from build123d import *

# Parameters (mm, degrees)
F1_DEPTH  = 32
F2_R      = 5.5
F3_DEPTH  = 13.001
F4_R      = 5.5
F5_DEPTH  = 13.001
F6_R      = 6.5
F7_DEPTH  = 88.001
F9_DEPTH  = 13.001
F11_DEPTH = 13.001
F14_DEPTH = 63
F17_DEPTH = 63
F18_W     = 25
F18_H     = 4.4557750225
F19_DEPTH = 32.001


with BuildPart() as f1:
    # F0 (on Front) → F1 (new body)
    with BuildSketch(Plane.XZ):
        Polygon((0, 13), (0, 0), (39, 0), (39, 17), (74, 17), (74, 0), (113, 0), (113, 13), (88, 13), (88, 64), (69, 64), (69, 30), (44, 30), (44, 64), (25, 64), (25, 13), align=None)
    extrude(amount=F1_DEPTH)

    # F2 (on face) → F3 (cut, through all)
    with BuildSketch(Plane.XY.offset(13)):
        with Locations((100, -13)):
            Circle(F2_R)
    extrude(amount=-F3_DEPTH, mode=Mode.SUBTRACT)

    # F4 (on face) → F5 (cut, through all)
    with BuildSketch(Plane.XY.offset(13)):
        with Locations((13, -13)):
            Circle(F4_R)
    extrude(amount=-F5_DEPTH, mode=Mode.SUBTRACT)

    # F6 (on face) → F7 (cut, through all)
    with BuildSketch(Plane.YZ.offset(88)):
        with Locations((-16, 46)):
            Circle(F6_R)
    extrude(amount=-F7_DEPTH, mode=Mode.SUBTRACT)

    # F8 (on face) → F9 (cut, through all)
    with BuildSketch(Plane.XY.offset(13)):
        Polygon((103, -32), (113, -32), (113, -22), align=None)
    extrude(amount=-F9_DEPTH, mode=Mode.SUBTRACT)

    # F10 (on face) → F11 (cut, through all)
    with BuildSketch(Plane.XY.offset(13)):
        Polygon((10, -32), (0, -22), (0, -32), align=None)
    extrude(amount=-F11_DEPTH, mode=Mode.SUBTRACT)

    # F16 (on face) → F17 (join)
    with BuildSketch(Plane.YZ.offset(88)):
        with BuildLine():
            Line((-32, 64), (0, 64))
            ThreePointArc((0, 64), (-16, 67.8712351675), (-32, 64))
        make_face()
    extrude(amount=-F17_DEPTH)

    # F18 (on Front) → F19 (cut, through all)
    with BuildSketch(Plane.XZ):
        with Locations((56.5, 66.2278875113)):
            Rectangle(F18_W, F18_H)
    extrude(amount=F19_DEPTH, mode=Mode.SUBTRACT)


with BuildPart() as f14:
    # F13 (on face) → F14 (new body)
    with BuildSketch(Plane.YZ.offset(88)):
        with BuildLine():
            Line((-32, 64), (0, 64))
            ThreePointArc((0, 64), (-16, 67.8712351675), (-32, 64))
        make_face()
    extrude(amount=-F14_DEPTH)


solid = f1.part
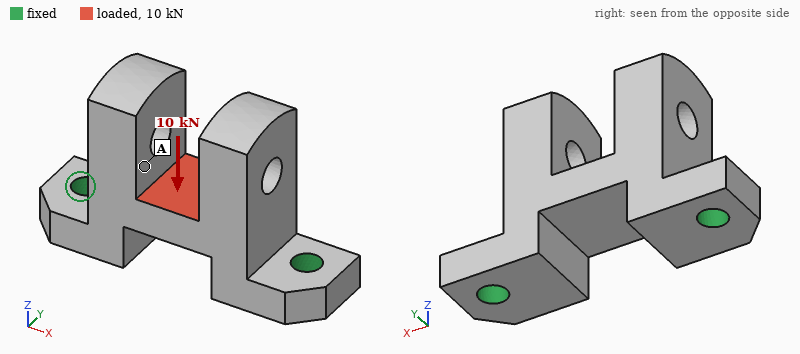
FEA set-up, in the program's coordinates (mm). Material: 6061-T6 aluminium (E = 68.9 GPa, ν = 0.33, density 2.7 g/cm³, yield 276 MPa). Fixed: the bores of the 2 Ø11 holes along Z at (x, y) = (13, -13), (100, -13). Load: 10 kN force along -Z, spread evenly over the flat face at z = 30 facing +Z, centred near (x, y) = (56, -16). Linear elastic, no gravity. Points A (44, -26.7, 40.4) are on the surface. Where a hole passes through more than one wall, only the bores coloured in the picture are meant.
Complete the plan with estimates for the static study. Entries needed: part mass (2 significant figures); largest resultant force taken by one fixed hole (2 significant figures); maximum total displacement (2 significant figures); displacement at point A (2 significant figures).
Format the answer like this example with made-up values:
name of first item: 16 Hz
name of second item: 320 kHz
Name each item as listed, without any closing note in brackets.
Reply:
part mass: 260 g
largest resultant force taken by one fixed hole: 7.4 kN
maximum total displacement: 54 µm
displacement at point A: 37 µm
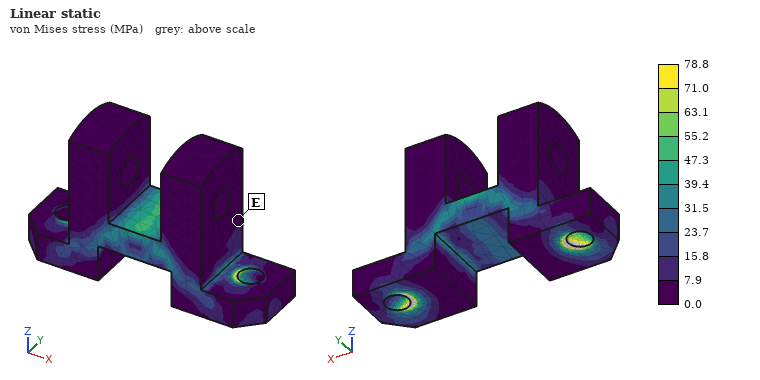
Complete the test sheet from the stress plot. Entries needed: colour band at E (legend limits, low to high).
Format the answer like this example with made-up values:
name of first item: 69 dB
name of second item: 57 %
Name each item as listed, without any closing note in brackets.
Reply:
colour band at E: 0.0 to 7.9 MPa
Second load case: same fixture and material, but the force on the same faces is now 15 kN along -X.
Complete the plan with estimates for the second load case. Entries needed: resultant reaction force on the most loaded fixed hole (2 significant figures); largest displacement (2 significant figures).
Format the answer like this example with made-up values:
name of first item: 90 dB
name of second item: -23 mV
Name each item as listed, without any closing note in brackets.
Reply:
resultant reaction force on the most loaded fixed hole: 8.7 kN
largest displacement: 41 µm
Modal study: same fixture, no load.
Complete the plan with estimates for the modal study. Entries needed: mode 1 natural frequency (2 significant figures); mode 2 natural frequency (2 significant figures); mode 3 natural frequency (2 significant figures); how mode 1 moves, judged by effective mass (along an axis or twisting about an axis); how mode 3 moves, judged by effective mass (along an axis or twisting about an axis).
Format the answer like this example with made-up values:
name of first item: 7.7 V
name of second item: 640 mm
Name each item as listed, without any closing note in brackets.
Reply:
mode 1 natural frequency: 2500 Hz
mode 2 natural frequency: 4100 Hz
mode 3 natural frequency: 4900 Hz
how mode 1 moves, judged by effective mass: along Y
how mode 3 moves, judged by effective mass: along X
